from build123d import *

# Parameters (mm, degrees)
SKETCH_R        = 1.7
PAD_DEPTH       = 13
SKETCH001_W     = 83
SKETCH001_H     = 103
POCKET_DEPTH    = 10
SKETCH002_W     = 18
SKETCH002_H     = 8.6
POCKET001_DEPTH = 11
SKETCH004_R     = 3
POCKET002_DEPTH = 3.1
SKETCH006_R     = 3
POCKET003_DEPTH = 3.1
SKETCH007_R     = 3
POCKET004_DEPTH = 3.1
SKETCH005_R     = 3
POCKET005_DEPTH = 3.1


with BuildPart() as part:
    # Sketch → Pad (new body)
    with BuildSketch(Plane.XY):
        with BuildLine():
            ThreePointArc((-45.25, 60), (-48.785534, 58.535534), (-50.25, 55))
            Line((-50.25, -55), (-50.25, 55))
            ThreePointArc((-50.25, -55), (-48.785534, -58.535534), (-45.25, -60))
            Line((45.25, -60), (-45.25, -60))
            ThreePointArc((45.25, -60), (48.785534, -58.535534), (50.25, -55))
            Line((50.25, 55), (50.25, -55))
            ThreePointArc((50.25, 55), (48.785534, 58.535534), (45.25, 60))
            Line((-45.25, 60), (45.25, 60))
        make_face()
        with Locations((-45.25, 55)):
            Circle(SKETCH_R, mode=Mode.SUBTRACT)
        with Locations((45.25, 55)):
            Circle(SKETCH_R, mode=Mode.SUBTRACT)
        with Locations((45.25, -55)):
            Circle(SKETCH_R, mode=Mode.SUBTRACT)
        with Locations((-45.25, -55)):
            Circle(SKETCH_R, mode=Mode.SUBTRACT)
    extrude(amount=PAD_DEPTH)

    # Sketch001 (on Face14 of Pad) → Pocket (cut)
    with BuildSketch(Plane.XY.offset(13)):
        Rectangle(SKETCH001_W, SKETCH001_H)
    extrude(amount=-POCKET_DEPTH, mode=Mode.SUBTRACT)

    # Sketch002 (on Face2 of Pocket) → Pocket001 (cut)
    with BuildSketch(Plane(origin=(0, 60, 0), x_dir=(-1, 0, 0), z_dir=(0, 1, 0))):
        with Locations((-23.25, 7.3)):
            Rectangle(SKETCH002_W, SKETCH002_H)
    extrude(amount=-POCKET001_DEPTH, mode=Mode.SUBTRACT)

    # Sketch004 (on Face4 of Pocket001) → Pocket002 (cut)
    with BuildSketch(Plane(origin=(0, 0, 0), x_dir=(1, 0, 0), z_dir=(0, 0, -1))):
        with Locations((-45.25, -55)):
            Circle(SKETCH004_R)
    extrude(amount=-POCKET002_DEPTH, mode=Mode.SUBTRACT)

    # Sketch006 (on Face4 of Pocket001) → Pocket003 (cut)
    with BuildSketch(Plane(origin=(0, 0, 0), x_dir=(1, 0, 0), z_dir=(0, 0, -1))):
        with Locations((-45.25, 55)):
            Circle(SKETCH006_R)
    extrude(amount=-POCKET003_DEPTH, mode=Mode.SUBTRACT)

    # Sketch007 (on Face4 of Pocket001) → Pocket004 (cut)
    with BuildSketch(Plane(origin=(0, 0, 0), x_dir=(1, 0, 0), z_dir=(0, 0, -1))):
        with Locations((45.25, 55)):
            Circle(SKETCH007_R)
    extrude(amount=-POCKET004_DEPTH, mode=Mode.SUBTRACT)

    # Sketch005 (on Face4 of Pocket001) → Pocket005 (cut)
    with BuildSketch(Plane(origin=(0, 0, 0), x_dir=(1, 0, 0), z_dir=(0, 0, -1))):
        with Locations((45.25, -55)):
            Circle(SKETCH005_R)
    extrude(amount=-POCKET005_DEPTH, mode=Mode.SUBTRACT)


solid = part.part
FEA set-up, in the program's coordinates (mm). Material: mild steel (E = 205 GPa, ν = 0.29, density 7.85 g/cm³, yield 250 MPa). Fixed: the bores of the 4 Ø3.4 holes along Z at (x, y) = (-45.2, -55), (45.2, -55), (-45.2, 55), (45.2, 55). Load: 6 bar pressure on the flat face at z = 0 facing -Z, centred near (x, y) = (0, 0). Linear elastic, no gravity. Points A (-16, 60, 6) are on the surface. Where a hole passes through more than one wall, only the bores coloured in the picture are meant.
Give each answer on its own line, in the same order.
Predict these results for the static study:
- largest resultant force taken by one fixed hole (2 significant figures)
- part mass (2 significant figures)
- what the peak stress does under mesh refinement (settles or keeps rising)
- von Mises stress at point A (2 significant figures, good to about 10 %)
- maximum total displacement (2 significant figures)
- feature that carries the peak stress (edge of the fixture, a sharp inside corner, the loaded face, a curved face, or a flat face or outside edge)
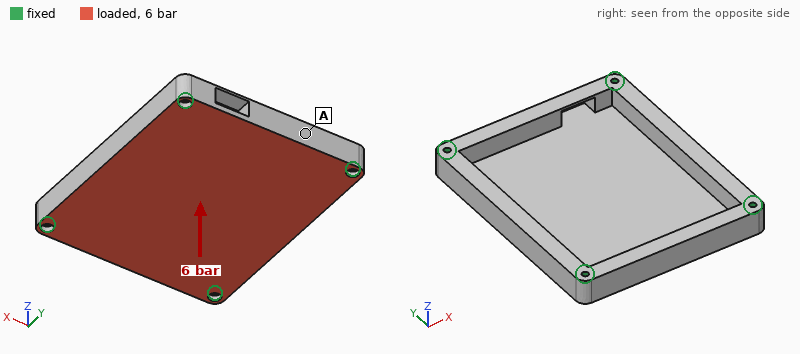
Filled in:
3.0 kN
540 g
keeps rising
24 MPa
0.19 mm
edge of the fixture
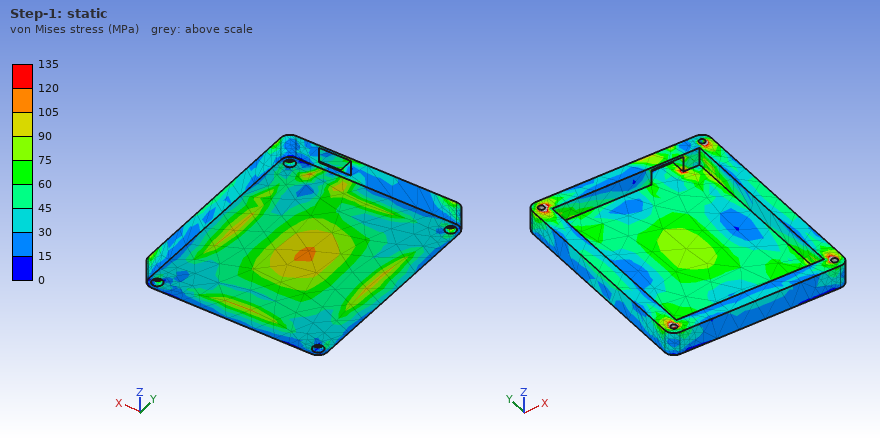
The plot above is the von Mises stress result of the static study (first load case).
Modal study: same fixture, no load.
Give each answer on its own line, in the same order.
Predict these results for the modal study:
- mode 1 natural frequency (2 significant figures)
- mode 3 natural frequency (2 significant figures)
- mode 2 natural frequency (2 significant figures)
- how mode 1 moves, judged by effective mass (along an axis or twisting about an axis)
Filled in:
2300 Hz
4100 Hz
4000 Hz
along Z
